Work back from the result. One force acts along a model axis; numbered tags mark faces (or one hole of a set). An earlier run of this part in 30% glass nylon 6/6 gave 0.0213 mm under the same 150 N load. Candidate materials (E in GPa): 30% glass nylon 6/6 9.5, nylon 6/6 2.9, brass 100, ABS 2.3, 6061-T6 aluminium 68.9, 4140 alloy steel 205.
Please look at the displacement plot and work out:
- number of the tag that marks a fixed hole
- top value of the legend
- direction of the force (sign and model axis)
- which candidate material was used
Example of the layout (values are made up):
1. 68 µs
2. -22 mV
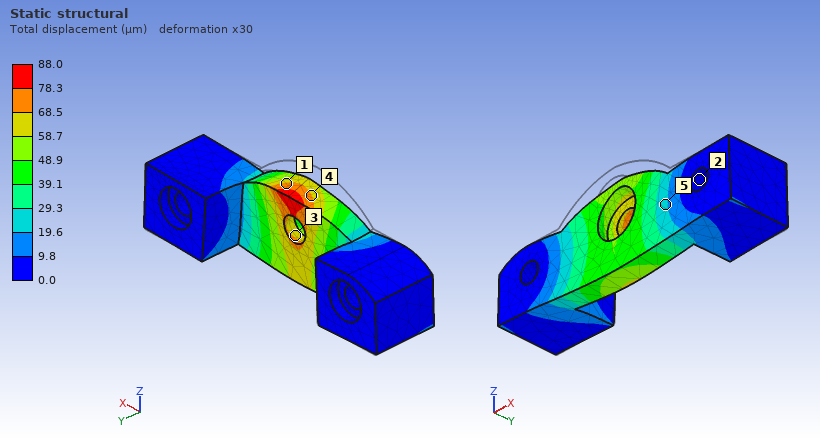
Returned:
1. 2
2. 88.0 µm
3. -Z
4. ABS
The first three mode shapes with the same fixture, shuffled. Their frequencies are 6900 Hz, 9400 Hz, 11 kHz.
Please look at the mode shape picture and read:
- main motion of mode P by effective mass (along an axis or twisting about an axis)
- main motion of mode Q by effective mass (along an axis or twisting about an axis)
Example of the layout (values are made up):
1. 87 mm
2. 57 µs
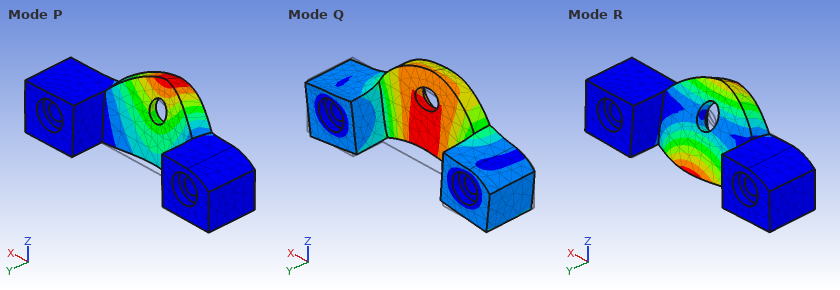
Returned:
1. along Y
2. along Z
